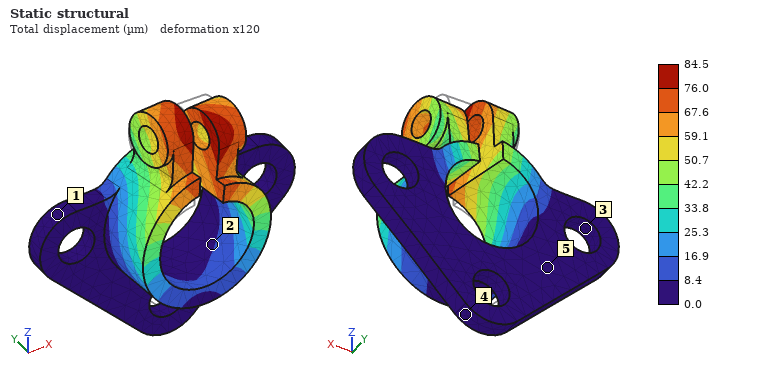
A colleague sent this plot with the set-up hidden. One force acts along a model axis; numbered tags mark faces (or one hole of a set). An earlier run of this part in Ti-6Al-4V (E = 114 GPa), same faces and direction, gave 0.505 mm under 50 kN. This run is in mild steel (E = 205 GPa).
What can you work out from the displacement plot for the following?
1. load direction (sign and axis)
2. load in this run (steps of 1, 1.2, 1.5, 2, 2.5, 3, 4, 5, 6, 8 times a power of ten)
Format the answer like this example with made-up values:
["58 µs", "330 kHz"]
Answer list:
["+X", "15 kN"]
